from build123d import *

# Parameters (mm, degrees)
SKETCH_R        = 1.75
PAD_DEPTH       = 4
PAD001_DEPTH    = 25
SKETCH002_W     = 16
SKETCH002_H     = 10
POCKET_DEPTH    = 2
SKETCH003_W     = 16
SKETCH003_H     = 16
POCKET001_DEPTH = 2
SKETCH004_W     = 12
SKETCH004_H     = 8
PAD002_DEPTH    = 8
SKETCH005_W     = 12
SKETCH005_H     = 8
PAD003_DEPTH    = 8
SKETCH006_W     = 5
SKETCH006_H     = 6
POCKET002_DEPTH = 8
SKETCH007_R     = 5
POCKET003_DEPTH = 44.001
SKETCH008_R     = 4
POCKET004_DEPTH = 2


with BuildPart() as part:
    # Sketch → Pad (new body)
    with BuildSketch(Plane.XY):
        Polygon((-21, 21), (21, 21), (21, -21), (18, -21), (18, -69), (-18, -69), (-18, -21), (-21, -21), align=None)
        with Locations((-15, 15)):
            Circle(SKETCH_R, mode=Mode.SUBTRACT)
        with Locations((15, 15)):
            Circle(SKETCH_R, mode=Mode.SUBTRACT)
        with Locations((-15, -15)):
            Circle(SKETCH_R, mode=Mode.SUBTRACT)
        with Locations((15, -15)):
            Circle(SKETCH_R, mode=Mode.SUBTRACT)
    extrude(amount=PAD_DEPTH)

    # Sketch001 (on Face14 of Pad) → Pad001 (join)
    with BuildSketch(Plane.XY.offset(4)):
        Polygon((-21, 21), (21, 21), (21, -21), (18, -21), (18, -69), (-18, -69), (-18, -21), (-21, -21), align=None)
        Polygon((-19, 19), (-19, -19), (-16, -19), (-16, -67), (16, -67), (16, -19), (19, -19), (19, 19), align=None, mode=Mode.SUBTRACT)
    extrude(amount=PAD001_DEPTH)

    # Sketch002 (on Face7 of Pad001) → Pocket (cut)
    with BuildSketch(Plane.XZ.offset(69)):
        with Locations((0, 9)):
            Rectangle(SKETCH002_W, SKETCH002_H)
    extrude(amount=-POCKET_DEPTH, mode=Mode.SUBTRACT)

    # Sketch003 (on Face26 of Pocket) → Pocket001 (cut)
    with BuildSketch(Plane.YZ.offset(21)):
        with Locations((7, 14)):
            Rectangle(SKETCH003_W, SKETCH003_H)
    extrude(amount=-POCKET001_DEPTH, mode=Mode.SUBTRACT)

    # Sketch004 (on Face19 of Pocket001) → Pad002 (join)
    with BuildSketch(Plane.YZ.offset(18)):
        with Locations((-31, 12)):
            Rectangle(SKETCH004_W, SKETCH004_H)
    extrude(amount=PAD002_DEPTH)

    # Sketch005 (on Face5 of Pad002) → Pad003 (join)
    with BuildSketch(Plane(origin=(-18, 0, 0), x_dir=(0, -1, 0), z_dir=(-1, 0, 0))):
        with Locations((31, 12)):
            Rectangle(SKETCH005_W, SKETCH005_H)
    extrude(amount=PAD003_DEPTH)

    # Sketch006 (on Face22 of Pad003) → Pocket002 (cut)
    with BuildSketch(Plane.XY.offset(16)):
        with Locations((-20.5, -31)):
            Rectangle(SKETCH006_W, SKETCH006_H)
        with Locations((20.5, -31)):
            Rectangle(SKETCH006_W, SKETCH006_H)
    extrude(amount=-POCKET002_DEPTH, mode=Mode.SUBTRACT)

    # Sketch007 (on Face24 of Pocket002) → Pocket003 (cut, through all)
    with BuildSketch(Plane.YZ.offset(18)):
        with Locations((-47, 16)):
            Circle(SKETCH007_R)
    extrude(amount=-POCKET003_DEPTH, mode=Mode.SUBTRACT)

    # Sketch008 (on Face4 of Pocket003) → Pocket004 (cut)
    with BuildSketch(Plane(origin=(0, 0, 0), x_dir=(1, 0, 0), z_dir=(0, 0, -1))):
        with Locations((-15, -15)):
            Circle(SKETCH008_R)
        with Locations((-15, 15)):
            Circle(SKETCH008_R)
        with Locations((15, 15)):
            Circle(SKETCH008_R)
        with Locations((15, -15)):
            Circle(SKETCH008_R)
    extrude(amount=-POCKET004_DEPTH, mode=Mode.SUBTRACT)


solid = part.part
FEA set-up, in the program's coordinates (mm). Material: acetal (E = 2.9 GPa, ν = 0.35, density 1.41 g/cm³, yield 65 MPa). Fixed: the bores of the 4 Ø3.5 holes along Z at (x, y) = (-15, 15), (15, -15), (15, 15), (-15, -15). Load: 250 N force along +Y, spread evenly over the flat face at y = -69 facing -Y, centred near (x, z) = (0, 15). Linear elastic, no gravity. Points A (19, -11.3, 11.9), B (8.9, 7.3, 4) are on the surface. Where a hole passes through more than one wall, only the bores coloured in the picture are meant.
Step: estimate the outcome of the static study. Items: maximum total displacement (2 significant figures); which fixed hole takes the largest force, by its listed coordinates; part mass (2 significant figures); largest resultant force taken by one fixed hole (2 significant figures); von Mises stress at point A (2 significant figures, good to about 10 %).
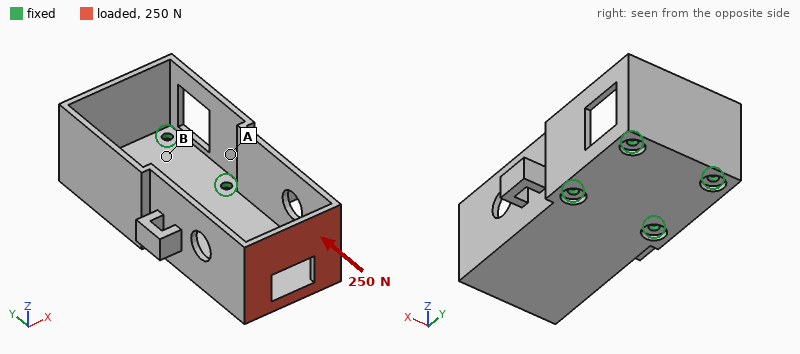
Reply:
1.2 mm
(15, -15)
37 g
110 N
4.5 MPa
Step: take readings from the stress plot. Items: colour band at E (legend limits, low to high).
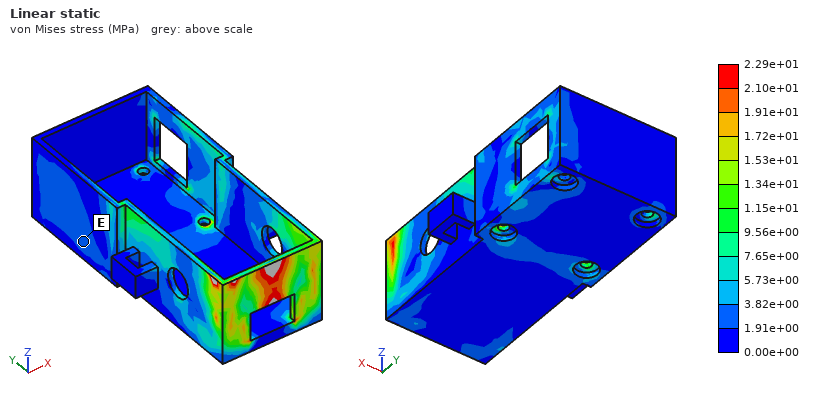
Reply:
1.91e+00 to 3.82e+00 MPa
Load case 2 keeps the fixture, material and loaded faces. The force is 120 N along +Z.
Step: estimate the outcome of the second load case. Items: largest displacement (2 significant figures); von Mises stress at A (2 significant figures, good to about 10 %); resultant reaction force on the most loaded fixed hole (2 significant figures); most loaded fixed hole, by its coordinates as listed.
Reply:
1.3 mm
8.8 MPa
170 N
(-15, -15)
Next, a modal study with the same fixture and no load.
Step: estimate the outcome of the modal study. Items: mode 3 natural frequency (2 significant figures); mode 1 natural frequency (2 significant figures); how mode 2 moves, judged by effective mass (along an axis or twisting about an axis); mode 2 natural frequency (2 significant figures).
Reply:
930 Hz
550 Hz
along Z
620 Hz
